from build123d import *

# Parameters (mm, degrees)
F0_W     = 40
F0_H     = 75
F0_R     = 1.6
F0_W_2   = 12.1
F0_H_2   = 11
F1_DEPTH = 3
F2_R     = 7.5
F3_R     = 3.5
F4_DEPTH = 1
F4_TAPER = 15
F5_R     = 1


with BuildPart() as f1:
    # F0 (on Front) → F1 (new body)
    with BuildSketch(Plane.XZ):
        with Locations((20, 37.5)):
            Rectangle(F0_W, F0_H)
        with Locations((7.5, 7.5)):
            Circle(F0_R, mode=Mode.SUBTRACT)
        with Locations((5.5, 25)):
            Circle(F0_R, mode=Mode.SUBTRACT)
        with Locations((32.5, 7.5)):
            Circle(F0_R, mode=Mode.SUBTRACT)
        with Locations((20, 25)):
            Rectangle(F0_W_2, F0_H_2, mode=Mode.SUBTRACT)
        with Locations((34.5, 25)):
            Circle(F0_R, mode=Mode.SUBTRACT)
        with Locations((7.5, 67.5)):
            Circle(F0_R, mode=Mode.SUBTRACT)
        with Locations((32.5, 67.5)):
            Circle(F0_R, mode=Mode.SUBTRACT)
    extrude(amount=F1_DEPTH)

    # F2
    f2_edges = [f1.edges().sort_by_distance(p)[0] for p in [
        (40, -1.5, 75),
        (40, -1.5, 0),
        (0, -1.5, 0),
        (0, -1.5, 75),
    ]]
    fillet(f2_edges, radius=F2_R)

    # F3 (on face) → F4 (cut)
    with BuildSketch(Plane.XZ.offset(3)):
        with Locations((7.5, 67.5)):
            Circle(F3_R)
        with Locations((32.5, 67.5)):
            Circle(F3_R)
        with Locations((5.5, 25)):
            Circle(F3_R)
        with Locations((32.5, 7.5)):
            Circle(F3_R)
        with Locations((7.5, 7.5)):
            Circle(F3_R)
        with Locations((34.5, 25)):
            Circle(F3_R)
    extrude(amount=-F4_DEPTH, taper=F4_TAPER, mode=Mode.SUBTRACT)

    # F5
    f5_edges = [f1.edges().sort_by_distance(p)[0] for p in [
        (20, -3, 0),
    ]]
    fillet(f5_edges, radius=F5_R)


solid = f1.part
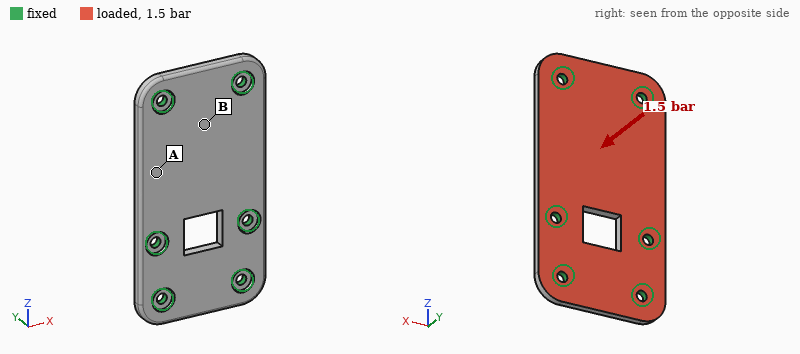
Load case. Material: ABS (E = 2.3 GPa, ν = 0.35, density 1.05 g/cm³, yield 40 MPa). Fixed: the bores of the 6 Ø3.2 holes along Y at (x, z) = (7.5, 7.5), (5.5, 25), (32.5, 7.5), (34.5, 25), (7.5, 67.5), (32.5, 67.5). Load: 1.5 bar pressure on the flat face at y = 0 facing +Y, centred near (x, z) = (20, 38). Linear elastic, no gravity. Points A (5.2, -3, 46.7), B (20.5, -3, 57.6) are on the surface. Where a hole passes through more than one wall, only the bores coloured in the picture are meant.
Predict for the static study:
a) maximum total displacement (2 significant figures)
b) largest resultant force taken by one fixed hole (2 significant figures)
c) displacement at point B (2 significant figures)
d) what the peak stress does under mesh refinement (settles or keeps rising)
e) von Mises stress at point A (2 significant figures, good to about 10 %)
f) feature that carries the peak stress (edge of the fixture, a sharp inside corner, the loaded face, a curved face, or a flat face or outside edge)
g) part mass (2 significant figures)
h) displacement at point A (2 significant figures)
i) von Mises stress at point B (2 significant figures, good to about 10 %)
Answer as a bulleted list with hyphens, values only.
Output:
- 0.39 mm
- 95 N
- 0.25 mm
- keeps rising
- 9.9 MPa
- edge of the fixture
- 8.5 g
- 0.37 mm
- 4.0 MPa
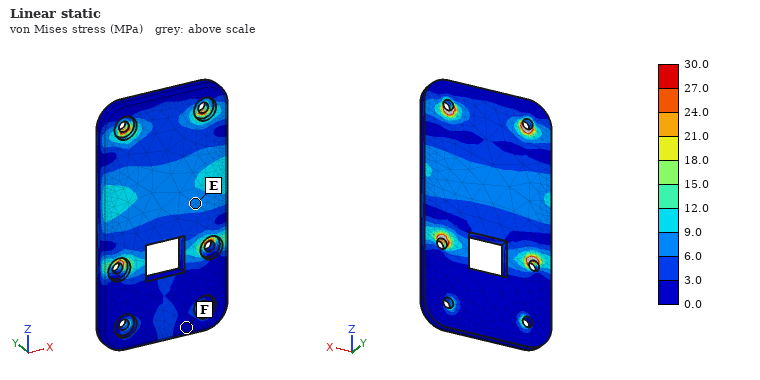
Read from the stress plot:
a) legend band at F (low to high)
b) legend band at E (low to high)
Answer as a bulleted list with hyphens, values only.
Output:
- 0.0 to 3.0 MPa
- 6.0 to 9.0 MPa
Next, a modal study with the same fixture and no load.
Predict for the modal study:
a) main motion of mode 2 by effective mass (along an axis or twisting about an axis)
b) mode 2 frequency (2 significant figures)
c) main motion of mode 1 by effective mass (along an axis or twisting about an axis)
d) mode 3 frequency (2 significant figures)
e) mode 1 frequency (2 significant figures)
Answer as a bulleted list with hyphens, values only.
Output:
- twisting about Z
- 2600 Hz
- along Y
- 4100 Hz
- 2000 Hz
